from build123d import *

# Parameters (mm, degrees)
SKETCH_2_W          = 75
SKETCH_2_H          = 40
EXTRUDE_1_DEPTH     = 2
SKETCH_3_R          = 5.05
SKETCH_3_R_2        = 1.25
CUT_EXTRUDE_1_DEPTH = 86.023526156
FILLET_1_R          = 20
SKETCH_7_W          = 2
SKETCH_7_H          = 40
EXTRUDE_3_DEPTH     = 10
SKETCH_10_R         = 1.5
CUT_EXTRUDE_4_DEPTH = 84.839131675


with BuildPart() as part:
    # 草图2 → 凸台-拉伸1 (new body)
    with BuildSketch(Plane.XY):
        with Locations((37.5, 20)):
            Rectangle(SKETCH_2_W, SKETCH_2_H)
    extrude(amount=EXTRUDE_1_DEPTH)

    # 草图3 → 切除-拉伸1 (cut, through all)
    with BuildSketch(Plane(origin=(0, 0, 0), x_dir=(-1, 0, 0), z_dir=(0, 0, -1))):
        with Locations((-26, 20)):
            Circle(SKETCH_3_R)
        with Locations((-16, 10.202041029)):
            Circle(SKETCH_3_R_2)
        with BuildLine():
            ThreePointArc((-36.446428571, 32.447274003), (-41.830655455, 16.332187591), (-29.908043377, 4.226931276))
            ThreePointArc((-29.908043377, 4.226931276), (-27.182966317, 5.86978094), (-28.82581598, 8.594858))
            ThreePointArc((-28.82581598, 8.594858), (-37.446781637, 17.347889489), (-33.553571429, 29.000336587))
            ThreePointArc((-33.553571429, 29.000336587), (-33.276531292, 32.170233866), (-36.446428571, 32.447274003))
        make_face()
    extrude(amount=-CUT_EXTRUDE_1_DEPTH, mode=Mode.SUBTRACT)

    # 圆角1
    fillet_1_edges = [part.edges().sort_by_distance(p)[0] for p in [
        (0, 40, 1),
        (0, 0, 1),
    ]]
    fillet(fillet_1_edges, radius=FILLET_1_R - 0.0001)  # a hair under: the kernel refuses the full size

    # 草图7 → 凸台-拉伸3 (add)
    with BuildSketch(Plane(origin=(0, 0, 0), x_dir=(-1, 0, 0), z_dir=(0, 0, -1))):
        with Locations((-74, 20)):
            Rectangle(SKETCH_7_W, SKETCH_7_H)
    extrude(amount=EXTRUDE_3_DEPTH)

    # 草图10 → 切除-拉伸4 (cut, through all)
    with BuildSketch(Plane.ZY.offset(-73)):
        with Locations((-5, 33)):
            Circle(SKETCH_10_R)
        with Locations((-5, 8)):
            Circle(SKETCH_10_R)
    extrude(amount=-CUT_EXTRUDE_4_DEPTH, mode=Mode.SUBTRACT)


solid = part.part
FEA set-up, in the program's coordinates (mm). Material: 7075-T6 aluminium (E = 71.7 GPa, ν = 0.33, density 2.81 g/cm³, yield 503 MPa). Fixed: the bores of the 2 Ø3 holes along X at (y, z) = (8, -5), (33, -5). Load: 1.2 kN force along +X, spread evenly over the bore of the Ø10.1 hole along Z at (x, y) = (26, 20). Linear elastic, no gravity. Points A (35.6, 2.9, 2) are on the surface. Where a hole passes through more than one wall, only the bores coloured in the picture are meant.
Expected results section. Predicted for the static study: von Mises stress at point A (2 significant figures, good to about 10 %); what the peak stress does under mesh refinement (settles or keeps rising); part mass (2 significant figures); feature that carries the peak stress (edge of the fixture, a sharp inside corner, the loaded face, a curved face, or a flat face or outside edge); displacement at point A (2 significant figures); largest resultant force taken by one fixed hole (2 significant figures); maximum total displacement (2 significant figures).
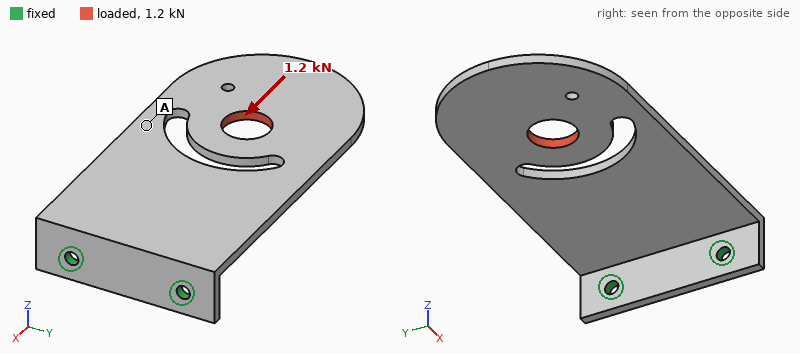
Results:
49 MPa
keeps rising
17 g
edge of the fixture
0.49 mm
620 N
0.92 mm
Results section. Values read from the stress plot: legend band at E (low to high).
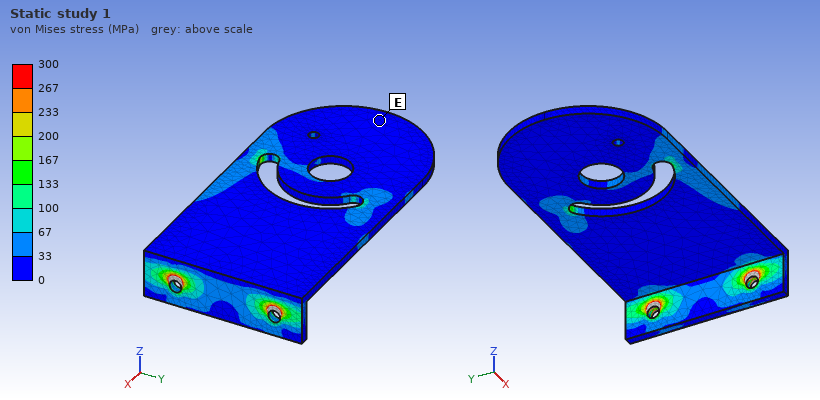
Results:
0 to 33 MPa
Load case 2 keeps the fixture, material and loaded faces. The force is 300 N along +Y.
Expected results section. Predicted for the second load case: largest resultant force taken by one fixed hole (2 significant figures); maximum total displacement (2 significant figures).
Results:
570 N
0.28 mm
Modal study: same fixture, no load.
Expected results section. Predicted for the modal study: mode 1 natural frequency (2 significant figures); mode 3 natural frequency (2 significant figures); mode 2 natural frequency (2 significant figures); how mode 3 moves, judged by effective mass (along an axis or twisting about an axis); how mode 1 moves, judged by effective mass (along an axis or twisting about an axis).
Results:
290 Hz
1500 Hz
1200 Hz
along Z
along Z
